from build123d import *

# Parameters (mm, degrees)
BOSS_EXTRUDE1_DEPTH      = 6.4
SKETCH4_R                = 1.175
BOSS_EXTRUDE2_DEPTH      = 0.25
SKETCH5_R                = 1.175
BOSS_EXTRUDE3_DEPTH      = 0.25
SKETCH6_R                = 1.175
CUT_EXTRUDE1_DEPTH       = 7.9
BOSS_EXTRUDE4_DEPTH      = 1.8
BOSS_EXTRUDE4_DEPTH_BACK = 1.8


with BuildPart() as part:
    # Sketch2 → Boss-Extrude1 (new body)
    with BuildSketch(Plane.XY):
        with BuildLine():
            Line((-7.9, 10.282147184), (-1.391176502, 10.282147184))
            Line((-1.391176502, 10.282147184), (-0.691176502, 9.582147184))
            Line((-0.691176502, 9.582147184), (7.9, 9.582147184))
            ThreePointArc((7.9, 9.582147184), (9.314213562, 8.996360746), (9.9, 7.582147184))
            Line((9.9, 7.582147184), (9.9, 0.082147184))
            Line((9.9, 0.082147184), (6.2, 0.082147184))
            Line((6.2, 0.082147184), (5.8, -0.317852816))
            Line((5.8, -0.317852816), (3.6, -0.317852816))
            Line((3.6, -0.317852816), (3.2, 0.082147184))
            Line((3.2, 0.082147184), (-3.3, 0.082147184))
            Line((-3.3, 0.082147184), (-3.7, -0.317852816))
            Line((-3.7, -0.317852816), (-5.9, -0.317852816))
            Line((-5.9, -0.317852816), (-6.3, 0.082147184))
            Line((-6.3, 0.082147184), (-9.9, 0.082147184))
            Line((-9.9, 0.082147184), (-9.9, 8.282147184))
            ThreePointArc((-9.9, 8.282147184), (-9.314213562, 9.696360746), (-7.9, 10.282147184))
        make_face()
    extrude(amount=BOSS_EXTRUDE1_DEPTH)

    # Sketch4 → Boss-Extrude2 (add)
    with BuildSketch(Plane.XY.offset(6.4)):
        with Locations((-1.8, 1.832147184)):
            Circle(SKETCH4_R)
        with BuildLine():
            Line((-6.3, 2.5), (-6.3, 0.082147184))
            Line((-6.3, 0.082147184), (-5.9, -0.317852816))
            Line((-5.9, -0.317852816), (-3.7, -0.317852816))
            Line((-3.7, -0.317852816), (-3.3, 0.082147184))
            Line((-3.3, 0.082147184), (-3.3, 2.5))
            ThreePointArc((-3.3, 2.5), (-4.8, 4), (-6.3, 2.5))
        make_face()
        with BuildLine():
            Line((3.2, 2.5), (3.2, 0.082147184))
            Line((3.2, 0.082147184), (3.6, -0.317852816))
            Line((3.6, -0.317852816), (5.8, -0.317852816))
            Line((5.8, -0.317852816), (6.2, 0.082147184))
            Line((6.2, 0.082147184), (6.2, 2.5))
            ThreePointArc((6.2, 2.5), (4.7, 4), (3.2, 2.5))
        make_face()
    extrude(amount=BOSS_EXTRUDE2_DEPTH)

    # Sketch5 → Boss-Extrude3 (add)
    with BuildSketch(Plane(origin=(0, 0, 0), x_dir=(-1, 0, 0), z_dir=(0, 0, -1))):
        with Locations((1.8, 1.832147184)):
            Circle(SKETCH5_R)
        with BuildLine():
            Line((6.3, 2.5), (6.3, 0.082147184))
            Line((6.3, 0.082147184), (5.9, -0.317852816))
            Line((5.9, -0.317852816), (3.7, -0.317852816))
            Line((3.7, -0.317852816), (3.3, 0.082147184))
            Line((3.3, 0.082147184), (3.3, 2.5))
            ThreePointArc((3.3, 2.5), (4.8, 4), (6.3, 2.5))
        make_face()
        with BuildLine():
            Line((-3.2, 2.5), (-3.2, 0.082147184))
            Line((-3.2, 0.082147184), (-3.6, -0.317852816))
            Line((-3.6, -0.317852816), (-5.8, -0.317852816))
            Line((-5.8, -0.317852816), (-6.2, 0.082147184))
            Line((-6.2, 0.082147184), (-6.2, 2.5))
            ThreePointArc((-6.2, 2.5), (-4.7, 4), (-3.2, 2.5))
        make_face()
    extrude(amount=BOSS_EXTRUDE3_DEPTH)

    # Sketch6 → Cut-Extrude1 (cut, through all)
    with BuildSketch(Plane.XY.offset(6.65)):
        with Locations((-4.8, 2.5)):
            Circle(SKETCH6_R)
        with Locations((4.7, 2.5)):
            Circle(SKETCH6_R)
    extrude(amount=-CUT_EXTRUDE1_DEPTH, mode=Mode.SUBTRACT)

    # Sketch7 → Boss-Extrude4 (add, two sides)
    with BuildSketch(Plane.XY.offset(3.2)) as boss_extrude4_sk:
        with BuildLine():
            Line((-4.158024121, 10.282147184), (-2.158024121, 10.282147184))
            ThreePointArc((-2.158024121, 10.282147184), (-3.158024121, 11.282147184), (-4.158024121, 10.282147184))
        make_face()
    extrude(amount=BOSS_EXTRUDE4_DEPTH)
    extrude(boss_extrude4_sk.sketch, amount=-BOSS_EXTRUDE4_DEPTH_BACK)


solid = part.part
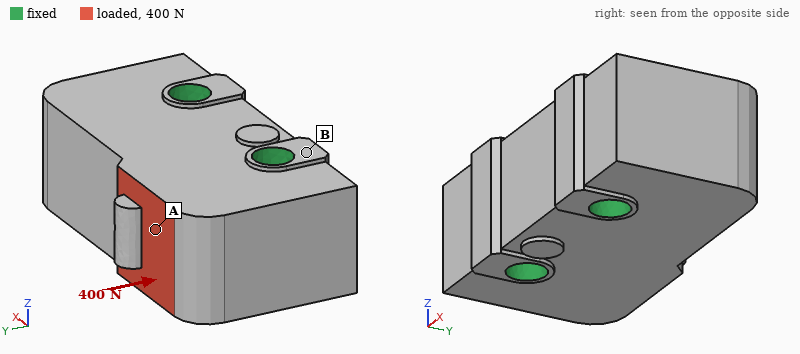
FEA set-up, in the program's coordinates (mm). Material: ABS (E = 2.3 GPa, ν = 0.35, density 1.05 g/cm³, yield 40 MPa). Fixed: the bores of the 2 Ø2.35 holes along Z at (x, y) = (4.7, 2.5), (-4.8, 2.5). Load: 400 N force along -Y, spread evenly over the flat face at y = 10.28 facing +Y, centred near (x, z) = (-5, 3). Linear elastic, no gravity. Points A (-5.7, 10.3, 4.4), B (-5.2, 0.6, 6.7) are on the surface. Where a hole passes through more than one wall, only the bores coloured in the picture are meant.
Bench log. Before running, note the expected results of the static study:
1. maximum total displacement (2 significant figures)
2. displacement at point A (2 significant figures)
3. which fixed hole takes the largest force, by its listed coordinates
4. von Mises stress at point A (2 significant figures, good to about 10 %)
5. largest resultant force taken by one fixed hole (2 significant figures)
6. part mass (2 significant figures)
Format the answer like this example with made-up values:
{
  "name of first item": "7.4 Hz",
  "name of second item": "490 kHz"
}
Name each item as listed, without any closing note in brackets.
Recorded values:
{
  "maximum total displacement": "41 µm",
  "displacement at point A": "38 µm",
  "which fixed hole takes the largest force, by its listed coordinates": "(-4.8, 2.5)",
  "von Mises stress at point A": "9.2 MPa",
  "largest resultant force taken by one fixed hole": "380 N",
  "part mass": "1.3 g"
}
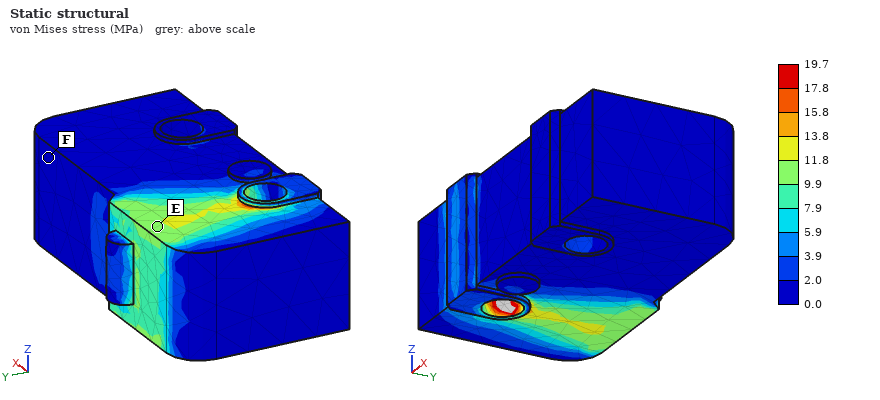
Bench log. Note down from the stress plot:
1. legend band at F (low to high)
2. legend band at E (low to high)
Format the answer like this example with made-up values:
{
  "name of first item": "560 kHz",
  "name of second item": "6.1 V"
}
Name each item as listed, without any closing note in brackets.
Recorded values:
{
  "legend band at F": "0.0 to 2.0 MPa",
  "legend band at E": "9.9 to 11.8 MPa"
}
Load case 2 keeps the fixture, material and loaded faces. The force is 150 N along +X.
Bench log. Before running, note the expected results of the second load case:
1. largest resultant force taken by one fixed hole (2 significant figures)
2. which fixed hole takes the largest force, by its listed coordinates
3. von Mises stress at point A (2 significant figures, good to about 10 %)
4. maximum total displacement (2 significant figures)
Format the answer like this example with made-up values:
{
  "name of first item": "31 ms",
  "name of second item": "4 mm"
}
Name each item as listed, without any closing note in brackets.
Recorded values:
{
  "largest resultant force taken by one fixed hole": "130 N",
  "which fixed hole takes the largest force, by its listed coordinates": "(4.7, 2.5)",
  "von Mises stress at point A": "8.6 MPa",
  "maximum total displacement": "38 µm"
}
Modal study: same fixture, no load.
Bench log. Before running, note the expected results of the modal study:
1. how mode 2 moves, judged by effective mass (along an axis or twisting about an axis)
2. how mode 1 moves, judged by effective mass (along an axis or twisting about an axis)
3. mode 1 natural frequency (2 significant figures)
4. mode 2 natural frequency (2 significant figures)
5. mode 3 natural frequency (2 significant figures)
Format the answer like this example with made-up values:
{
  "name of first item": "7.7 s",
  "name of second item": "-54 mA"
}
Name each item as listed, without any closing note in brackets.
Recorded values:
{
  "how mode 2 moves, judged by effective mass": "along X",
  "how mode 1 moves, judged by effective mass": "along Z",
  "mode 1 natural frequency": "18 kHz",
  "mode 2 natural frequency": "21 kHz",
  "mode 3 natural frequency": "22 kHz"
}
